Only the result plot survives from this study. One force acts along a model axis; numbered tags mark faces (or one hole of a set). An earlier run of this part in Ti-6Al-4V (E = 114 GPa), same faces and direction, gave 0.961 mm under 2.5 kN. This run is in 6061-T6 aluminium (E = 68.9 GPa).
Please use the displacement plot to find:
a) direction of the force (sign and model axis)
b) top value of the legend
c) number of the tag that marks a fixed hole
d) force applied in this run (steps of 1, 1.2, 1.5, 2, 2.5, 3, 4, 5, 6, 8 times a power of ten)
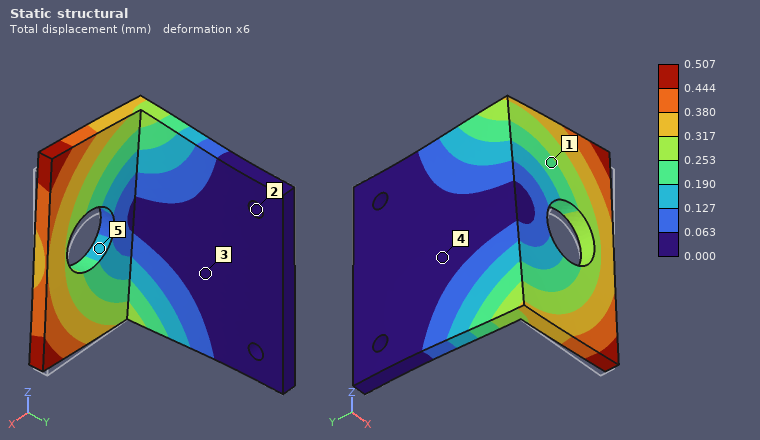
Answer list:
+Z
0.507 mm
2
800 N
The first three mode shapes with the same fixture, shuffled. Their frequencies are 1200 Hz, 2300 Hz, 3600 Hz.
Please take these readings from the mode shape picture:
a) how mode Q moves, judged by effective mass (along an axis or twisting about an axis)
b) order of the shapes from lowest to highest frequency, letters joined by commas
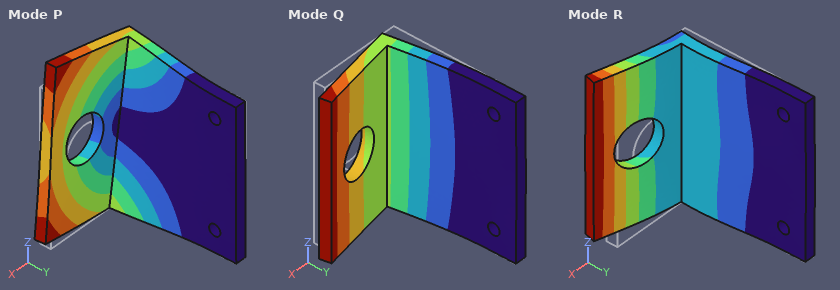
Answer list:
along X
Q, P, R
